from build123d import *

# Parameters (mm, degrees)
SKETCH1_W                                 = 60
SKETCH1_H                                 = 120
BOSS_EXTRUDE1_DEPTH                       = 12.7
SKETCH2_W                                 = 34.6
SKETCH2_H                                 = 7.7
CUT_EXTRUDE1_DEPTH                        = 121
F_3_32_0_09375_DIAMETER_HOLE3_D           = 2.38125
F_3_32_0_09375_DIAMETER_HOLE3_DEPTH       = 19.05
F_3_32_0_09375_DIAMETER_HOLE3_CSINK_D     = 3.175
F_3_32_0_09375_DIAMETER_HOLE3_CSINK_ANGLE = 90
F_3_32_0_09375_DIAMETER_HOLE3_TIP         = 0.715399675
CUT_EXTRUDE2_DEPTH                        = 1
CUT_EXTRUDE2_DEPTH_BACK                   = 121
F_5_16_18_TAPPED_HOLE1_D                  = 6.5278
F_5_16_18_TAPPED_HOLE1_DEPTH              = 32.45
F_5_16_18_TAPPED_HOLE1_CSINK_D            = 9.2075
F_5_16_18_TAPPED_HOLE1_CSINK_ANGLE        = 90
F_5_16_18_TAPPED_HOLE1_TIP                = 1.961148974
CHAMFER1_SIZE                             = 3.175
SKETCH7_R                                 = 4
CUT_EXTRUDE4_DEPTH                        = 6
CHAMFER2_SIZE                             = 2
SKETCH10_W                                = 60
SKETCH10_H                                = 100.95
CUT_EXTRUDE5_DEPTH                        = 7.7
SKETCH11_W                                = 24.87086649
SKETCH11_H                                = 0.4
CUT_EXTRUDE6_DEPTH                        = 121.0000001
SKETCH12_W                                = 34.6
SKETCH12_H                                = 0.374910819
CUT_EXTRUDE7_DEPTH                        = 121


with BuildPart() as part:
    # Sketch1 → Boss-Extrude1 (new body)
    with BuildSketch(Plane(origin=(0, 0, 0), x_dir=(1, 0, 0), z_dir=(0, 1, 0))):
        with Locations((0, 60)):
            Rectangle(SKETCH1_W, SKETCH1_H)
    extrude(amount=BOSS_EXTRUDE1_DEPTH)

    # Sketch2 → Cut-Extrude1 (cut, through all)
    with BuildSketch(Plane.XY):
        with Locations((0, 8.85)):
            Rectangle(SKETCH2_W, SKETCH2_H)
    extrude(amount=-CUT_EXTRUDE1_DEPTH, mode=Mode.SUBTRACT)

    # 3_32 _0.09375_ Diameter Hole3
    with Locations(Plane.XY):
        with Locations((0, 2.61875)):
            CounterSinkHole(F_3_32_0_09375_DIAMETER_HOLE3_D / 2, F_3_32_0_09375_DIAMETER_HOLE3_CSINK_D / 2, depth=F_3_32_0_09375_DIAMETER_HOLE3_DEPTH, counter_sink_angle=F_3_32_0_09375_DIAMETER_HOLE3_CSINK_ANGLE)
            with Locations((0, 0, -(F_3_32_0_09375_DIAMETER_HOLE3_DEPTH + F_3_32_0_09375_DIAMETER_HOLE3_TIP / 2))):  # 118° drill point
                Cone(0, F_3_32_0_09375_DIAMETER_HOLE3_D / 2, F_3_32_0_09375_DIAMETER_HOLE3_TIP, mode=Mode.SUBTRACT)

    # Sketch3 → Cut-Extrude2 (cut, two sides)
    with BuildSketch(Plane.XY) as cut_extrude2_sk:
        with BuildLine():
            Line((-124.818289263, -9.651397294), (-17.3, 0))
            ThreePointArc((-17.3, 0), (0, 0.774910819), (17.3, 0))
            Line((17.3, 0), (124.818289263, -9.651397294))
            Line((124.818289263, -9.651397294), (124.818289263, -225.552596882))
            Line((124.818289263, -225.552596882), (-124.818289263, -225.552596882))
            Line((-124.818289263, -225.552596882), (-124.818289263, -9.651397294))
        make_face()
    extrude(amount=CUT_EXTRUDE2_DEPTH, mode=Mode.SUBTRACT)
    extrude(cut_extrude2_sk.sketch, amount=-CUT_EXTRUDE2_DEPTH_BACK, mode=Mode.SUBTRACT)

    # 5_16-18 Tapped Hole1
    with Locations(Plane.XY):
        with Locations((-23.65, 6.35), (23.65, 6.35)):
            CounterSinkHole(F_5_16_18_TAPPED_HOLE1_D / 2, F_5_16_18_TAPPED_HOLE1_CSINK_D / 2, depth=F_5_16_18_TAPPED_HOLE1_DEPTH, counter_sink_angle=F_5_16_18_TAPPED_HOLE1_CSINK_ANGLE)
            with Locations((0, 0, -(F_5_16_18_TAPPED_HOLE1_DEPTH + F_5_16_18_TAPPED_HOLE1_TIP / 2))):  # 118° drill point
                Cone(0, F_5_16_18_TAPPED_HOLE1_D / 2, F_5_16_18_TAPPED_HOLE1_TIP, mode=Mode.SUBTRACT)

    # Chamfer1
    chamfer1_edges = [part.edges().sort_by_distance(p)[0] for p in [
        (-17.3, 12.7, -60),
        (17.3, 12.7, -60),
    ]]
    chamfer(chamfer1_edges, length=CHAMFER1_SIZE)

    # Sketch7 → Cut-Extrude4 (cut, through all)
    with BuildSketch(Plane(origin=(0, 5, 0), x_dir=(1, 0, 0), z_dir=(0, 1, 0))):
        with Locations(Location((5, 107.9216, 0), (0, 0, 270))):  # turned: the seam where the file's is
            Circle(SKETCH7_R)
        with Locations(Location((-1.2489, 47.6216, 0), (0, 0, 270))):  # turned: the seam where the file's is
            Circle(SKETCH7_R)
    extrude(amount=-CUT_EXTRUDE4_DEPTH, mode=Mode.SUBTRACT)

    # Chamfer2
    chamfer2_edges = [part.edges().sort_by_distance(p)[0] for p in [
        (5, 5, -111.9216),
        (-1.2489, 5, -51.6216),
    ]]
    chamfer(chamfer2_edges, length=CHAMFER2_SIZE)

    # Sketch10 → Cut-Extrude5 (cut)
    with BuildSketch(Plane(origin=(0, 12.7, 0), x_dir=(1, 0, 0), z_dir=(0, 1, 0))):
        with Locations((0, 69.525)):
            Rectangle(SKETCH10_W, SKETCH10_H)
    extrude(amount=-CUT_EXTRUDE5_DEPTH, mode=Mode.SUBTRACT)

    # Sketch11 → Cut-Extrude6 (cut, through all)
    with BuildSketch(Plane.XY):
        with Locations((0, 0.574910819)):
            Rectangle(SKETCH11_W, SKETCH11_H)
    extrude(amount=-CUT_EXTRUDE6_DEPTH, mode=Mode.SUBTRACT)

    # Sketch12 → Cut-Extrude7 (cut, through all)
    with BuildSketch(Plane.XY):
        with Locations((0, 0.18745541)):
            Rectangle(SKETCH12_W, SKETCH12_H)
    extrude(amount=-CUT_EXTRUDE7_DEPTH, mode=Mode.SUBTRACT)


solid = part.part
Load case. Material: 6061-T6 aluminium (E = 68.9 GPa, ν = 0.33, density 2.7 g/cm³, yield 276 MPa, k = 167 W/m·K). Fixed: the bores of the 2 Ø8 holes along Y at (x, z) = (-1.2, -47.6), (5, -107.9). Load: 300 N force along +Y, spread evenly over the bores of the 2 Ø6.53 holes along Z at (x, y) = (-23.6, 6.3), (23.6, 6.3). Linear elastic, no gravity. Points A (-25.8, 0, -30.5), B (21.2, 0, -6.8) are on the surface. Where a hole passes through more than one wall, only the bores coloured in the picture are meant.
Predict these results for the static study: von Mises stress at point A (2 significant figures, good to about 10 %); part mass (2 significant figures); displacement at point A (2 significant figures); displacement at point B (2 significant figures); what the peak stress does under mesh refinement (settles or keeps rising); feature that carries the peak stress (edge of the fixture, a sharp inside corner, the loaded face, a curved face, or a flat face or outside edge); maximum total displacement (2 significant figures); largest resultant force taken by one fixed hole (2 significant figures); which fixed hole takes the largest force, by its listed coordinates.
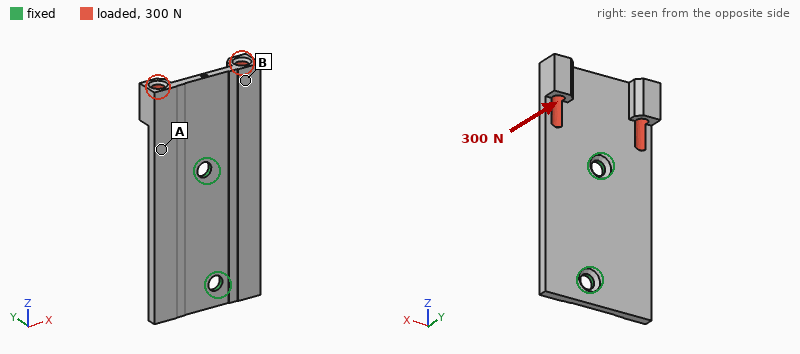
24 MPa
93 g
0.074 mm
0.24 mm
keeps rising
edge of the fixture
0.30 mm
400 N
(-1.2, -47.6)
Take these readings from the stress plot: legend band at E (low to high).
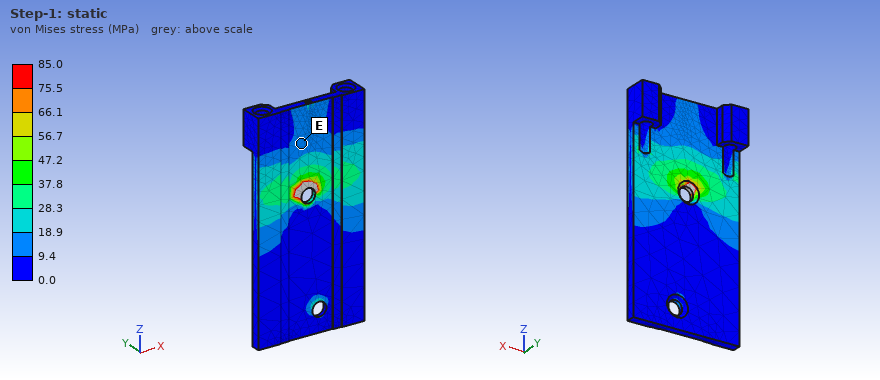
9.4 to 18.9 MPa
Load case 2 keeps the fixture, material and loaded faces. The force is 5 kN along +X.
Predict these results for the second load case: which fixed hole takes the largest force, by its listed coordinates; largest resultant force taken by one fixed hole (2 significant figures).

(-1.2, -47.6)
7.4 kN
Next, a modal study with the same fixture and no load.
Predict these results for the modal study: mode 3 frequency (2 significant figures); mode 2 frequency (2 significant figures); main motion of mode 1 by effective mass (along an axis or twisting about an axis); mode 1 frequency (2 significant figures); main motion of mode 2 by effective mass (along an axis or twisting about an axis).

2600 Hz
1600 Hz
along Y
1200 Hz
twisting about Z
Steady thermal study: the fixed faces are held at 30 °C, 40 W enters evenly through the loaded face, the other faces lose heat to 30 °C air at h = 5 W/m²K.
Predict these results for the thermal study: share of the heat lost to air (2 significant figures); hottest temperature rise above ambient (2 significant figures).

3.2 %
42 K
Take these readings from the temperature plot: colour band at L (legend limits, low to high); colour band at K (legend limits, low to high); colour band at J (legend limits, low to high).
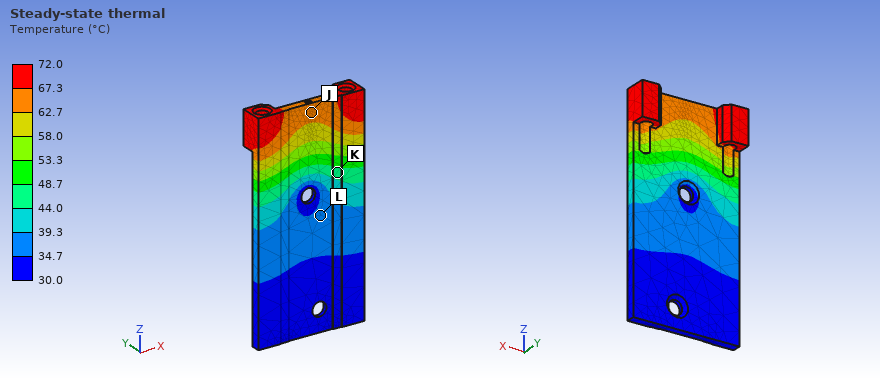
34.7 to 39.3 °C
44.0 to 48.7 °C
62.7 to 67.3 °C
